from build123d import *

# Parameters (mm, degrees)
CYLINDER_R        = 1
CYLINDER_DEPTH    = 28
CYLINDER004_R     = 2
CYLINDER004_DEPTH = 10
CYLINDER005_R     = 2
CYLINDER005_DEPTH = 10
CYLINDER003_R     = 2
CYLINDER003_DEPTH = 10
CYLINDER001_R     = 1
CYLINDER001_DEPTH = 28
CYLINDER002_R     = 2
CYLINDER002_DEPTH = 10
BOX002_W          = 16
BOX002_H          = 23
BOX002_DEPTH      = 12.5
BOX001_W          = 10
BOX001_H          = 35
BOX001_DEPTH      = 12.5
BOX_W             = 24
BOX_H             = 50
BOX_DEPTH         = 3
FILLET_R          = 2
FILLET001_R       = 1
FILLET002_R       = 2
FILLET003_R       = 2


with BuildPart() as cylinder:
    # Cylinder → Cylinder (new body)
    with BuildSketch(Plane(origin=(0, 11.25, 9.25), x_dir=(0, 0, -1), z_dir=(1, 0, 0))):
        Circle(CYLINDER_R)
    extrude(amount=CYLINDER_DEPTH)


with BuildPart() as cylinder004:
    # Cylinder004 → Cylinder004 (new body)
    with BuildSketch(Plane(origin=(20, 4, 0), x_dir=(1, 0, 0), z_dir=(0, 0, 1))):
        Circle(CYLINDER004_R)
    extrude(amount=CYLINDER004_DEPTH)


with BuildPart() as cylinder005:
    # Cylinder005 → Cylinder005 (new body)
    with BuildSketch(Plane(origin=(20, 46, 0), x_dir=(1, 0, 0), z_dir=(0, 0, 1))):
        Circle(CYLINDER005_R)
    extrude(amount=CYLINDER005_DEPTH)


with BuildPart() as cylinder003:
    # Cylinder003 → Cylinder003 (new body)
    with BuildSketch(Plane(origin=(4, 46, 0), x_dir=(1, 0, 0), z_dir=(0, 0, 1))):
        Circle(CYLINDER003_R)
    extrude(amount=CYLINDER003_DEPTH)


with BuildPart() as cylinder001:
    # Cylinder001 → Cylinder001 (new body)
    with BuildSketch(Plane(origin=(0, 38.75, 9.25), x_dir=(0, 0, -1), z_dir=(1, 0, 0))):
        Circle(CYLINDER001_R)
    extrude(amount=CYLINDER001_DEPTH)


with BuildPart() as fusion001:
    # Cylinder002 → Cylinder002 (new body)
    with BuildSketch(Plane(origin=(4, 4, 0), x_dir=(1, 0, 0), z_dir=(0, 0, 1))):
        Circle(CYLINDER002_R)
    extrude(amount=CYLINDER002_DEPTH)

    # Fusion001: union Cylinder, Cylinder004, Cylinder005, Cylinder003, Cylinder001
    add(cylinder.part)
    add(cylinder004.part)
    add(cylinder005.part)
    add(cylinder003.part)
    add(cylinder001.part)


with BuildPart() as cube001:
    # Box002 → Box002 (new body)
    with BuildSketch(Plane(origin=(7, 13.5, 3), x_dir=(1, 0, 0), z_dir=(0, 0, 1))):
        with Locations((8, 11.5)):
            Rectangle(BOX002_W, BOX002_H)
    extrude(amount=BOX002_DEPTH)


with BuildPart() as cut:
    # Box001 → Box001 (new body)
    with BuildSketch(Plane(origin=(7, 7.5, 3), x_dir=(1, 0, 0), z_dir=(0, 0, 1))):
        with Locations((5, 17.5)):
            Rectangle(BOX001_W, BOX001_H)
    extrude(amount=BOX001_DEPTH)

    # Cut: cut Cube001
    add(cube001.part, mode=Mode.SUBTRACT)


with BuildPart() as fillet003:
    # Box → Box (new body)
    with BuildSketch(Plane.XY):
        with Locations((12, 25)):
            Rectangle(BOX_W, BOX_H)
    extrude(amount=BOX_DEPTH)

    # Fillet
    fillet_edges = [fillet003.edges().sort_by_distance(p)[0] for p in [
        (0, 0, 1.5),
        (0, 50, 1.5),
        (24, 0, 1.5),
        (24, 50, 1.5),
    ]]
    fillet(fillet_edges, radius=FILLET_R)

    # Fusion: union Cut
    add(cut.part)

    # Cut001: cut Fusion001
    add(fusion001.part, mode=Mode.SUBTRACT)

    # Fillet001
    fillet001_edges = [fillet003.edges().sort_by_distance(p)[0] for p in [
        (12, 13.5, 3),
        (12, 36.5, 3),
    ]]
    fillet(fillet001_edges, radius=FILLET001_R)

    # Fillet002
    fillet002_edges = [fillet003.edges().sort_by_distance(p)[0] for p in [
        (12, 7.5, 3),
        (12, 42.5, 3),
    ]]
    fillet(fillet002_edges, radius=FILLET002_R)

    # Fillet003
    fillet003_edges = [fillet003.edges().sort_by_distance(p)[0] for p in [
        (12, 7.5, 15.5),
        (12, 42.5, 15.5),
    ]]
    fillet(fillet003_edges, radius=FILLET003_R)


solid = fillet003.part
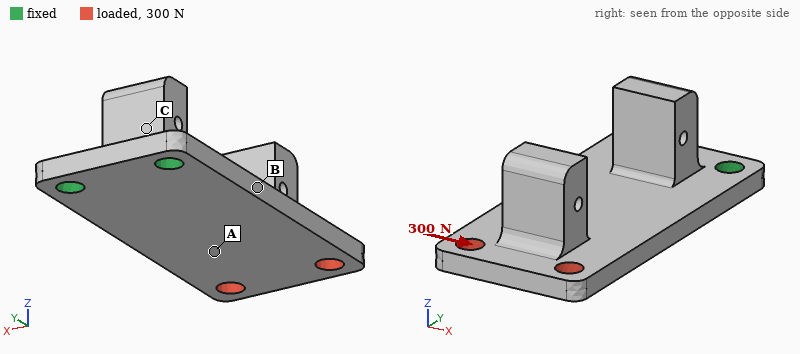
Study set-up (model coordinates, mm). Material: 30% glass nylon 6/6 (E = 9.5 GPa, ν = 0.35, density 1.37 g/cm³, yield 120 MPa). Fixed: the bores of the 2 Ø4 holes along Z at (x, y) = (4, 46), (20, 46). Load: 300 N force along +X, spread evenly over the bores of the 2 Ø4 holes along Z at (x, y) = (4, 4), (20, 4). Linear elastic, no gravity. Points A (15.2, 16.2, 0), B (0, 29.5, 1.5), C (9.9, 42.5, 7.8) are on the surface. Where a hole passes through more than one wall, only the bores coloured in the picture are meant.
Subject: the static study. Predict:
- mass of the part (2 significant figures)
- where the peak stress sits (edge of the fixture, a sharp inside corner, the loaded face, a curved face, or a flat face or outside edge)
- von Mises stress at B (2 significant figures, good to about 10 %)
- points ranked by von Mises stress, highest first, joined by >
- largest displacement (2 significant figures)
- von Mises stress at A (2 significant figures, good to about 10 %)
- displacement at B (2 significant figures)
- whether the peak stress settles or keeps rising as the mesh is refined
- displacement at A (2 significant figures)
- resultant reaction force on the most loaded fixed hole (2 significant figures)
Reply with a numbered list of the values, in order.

1. 6.7 g
2. edge of the fixture
3. 27 MPa
4. B > A > C
5. 0.32 mm
6. 11 MPa
7. 0.090 mm
8. keeps rising
9. 0.16 mm
10. 730 N
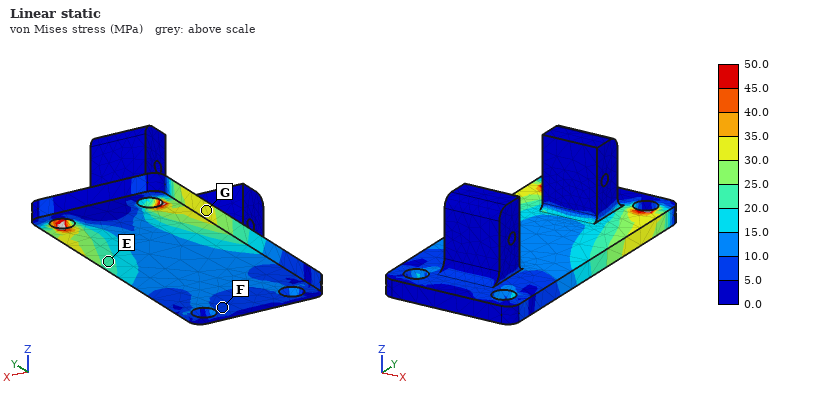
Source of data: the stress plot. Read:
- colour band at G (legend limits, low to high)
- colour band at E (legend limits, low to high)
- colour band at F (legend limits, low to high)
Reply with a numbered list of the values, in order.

1. 30.0 to 35.0 MPa
2. 20.0 to 25.0 MPa
3. 5.0 to 10.0 MPa
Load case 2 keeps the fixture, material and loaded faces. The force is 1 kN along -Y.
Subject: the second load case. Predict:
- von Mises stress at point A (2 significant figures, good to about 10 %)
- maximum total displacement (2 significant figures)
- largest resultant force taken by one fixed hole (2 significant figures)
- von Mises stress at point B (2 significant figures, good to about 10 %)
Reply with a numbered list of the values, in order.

1. 12 MPa
2. 99 µm
3. 510 N
4. 14 MPa
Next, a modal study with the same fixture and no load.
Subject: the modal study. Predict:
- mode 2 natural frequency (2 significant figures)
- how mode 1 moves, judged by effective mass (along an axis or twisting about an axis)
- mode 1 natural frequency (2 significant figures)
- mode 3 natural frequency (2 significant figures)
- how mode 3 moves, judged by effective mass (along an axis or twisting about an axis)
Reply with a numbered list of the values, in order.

1. 2100 Hz
2. along Z
3. 580 Hz
4. 3100 Hz
5. along Z
